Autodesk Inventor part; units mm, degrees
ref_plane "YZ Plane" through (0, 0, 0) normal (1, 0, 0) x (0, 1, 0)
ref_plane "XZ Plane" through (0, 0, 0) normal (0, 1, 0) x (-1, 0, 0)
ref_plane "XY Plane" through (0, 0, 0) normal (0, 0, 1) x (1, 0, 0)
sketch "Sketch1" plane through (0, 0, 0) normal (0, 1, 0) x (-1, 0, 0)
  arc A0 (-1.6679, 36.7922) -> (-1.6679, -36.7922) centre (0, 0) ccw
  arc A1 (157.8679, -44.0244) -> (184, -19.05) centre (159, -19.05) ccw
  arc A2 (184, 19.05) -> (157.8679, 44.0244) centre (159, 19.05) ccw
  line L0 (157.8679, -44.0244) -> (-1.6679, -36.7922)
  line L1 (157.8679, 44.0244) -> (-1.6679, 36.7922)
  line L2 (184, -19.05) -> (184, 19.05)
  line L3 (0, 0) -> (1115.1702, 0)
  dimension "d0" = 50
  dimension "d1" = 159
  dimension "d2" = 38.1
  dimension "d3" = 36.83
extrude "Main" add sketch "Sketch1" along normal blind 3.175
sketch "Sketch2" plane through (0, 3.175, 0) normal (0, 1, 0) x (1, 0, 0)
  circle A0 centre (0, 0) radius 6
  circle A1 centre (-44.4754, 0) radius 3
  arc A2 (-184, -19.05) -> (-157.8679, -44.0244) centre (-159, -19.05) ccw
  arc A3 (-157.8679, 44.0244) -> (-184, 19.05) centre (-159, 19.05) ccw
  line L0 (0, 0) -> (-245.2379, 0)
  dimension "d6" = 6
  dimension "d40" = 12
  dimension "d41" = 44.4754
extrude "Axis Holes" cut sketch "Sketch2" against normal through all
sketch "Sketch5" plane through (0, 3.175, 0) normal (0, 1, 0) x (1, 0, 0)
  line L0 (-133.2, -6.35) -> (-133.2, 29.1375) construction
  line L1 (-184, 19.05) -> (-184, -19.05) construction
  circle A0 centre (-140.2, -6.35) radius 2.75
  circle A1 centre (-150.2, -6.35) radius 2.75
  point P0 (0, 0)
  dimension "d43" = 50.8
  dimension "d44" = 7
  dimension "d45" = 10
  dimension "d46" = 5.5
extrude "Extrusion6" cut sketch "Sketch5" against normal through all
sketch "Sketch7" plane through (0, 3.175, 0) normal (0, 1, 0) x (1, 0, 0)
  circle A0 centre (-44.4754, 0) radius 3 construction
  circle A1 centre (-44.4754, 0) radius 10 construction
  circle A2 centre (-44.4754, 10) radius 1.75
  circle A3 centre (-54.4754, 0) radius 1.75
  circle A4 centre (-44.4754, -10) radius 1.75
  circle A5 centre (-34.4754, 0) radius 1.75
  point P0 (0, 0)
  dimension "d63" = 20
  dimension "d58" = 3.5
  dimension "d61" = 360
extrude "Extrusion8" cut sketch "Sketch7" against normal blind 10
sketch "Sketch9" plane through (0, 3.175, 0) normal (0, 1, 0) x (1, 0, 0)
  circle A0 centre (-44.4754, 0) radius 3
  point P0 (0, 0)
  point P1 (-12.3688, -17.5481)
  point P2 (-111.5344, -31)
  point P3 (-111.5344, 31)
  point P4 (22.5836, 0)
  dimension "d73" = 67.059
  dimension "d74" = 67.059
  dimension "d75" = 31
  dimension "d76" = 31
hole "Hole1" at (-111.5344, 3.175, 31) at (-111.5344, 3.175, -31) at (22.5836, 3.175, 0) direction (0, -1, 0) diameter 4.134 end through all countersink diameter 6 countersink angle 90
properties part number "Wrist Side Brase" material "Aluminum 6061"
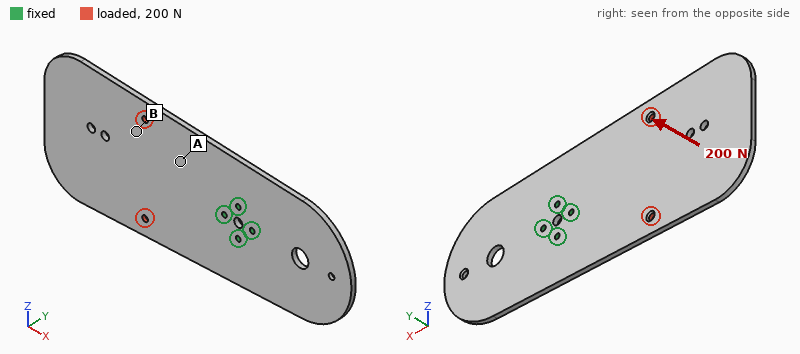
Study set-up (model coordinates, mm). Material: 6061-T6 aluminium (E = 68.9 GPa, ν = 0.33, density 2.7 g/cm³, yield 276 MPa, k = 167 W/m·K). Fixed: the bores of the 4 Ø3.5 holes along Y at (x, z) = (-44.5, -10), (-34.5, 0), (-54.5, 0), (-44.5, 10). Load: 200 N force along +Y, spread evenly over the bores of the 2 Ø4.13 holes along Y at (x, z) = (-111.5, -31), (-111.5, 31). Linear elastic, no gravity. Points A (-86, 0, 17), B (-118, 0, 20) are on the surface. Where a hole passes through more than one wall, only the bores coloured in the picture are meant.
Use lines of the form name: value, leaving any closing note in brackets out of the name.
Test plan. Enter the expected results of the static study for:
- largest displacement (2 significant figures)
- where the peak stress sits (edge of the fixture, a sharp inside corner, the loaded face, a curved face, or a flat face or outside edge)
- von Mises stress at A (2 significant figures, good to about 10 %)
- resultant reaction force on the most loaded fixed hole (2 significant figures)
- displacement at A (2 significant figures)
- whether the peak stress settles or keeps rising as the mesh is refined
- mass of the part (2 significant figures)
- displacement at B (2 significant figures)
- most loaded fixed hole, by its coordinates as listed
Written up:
largest displacement: 2.7 mm
where the peak stress sits: edge of the fixture
von Mises stress at A: 33 MPa
resultant reaction force on the most loaded fixed hole: 600 N
displacement at A: 0.44 mm
whether the peak stress settles or keeps rising as the mesh is refined: keeps rising
mass of the part: 140 g
displacement at B: 1.2 mm
most loaded fixed hole, by its coordinates as listed: (-54.5, 0)
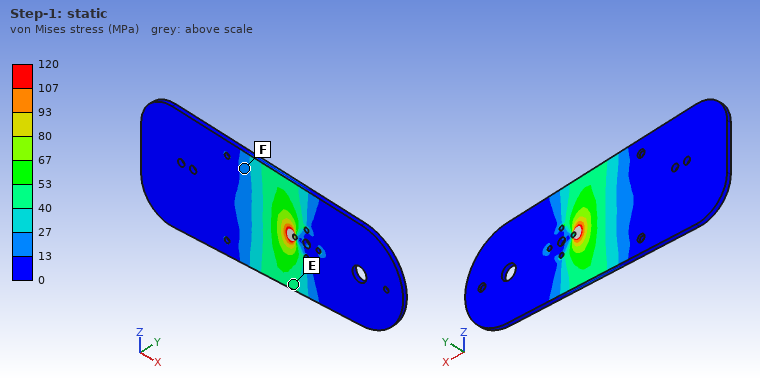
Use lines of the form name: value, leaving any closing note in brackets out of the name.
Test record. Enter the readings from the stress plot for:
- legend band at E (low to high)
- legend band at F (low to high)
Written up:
legend band at E: 40 to 53 MPa
legend band at F: 13 to 27 MPa
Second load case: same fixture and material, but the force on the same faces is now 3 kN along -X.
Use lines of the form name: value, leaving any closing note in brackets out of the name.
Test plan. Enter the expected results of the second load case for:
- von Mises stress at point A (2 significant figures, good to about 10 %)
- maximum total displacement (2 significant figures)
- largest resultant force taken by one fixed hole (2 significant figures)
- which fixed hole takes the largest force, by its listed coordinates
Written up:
von Mises stress at point A: 21 MPa
maximum total displacement: 0.57 mm
largest resultant force taken by one fixed hole: 960 N
which fixed hole takes the largest force, by its listed coordinates: (-54.5, 0)
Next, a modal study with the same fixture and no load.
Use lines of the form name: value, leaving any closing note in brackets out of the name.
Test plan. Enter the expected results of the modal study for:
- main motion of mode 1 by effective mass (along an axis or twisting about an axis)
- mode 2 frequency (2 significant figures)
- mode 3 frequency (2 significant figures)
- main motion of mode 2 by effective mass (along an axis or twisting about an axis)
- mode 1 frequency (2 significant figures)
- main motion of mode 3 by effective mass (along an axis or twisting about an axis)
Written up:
main motion of mode 1 by effective mass: along Y
mode 2 frequency: 450 Hz
mode 3 frequency: 560 Hz
main motion of mode 2 by effective mass: twisting about X
mode 1 frequency: 150 Hz
main motion of mode 3 by effective mass: along Y
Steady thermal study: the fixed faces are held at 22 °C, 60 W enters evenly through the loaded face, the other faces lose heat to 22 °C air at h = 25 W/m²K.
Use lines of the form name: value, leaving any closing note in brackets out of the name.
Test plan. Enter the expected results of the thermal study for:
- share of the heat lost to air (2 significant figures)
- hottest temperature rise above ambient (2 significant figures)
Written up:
share of the heat lost to air: 44 %
hottest temperature rise above ambient: 78 K
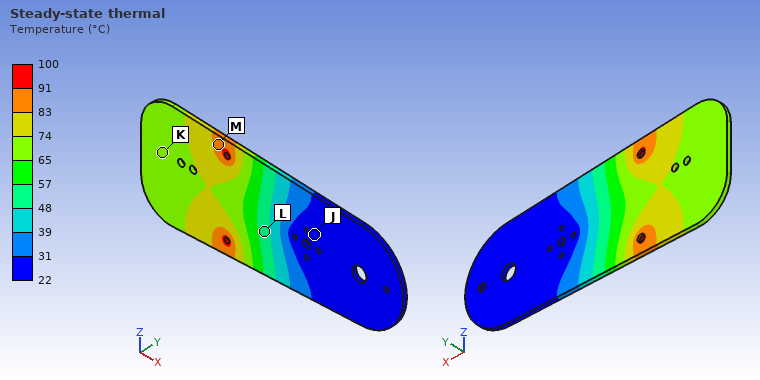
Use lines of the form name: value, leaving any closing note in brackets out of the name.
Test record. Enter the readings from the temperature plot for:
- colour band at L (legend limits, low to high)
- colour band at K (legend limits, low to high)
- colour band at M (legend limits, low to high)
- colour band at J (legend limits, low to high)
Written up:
colour band at L: 48 to 57 °C
colour band at K: 65 to 74 °C
colour band at M: 83 to 91 °C
colour band at J: 22 to 31 °C
